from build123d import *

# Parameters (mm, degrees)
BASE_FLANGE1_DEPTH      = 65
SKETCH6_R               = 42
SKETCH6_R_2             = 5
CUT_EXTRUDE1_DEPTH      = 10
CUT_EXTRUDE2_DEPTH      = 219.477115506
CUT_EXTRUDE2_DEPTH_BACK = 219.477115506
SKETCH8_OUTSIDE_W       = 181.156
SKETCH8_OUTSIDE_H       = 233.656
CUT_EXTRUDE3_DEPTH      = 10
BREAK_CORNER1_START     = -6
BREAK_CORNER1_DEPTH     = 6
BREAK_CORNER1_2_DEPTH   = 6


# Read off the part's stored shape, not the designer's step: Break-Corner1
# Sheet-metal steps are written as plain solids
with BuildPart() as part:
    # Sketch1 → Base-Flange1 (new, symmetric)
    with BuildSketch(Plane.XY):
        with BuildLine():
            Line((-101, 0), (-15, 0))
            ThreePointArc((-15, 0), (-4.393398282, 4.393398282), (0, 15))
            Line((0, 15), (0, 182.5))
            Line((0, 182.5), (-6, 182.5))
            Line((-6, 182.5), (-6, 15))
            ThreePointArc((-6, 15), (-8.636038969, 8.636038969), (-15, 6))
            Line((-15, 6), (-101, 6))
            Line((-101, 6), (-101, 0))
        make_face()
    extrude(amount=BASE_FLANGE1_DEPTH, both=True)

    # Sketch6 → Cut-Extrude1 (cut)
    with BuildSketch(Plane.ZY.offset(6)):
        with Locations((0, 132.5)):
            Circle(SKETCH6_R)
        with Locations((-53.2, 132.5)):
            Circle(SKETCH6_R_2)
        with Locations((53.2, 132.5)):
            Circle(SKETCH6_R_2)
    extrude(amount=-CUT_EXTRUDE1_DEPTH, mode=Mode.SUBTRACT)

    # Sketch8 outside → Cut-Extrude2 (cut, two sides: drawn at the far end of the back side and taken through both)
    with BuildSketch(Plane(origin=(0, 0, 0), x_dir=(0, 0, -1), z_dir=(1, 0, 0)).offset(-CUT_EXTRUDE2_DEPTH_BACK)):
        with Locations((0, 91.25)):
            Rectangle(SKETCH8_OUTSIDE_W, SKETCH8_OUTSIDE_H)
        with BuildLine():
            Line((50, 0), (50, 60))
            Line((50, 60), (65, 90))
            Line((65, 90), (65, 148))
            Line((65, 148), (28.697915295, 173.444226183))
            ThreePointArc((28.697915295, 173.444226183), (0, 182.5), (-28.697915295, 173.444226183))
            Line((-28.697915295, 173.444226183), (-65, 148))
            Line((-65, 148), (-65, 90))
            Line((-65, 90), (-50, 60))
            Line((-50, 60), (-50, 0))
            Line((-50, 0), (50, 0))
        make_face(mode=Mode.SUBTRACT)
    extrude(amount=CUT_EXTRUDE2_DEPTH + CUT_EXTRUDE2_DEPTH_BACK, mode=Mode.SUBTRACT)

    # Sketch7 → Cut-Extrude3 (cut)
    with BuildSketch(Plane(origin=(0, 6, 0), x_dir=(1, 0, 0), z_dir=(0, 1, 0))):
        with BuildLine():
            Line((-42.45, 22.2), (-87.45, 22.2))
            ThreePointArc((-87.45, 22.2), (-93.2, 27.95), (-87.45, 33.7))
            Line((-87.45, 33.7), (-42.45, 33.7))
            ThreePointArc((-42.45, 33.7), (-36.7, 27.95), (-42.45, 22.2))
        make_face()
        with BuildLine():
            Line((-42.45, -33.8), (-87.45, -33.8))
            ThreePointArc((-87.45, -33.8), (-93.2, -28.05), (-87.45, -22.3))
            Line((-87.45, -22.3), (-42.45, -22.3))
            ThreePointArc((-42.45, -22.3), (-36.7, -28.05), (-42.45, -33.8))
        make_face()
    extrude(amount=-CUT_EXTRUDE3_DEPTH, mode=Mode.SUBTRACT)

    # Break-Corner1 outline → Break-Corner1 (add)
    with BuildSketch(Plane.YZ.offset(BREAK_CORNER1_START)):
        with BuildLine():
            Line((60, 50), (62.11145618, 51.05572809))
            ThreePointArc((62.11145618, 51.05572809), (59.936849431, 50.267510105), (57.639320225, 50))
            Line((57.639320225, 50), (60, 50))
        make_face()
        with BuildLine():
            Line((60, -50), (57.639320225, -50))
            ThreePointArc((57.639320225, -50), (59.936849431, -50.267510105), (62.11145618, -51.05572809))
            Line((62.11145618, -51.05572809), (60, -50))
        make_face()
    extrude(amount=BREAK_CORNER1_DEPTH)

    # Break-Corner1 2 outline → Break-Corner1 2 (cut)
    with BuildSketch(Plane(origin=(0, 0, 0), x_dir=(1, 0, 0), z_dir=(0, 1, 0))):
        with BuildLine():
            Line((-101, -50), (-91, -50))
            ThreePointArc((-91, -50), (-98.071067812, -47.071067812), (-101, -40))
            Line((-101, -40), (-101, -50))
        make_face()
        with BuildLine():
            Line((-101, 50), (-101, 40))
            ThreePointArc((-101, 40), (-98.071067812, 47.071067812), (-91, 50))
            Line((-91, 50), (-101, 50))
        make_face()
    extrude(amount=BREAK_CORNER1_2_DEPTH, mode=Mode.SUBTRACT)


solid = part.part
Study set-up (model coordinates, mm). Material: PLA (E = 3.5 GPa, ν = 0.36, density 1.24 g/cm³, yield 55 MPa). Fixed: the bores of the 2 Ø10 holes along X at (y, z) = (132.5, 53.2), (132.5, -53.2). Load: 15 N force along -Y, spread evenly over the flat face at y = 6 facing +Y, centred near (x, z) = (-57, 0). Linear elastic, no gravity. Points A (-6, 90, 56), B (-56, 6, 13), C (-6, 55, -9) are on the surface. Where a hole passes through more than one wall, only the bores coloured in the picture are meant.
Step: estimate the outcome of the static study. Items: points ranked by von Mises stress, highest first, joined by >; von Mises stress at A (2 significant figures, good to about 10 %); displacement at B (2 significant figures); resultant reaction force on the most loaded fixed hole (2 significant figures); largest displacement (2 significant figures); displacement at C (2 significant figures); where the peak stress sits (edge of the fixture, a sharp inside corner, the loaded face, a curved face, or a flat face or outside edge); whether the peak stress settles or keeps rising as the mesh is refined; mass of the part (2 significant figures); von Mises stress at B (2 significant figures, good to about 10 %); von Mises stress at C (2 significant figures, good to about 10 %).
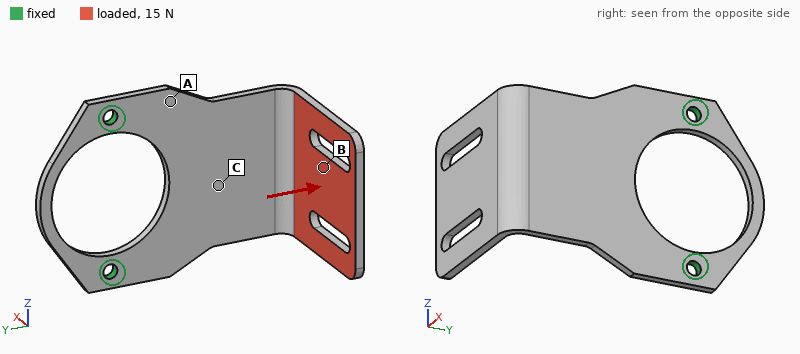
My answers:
A > C > B
1.6 MPa
1.8 mm
7.9 N
2.7 mm
0.60 mm
edge of the fixture
keeps rising
160 g
0.37 MPa
1.1 MPa
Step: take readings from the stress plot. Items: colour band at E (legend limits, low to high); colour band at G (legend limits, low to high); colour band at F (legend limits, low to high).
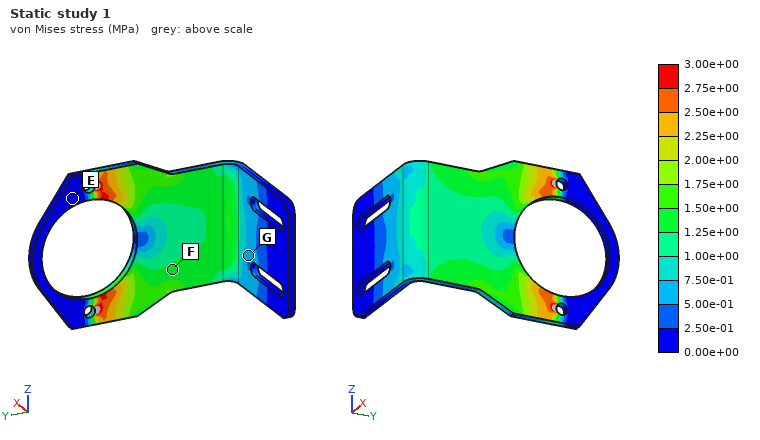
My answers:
0.00e+00 to 2.50e-01 MPa
5.00e-01 to 7.50e-01 MPa
1.25e+00 to 1.50e+00 MPa
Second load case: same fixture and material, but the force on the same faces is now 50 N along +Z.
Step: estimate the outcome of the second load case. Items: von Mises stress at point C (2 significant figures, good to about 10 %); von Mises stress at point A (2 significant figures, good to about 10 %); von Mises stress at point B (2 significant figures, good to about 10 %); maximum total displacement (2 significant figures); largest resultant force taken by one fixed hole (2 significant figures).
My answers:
3.6 MPa
2.1 MPa
0.59 MPa
2.8 mm
63 N
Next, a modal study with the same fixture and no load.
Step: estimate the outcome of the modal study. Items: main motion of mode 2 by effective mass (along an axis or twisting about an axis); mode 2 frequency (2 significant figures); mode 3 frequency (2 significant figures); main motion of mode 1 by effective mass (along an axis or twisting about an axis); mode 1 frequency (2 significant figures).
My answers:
along Z
98 Hz
140 Hz
along X
37 Hz
